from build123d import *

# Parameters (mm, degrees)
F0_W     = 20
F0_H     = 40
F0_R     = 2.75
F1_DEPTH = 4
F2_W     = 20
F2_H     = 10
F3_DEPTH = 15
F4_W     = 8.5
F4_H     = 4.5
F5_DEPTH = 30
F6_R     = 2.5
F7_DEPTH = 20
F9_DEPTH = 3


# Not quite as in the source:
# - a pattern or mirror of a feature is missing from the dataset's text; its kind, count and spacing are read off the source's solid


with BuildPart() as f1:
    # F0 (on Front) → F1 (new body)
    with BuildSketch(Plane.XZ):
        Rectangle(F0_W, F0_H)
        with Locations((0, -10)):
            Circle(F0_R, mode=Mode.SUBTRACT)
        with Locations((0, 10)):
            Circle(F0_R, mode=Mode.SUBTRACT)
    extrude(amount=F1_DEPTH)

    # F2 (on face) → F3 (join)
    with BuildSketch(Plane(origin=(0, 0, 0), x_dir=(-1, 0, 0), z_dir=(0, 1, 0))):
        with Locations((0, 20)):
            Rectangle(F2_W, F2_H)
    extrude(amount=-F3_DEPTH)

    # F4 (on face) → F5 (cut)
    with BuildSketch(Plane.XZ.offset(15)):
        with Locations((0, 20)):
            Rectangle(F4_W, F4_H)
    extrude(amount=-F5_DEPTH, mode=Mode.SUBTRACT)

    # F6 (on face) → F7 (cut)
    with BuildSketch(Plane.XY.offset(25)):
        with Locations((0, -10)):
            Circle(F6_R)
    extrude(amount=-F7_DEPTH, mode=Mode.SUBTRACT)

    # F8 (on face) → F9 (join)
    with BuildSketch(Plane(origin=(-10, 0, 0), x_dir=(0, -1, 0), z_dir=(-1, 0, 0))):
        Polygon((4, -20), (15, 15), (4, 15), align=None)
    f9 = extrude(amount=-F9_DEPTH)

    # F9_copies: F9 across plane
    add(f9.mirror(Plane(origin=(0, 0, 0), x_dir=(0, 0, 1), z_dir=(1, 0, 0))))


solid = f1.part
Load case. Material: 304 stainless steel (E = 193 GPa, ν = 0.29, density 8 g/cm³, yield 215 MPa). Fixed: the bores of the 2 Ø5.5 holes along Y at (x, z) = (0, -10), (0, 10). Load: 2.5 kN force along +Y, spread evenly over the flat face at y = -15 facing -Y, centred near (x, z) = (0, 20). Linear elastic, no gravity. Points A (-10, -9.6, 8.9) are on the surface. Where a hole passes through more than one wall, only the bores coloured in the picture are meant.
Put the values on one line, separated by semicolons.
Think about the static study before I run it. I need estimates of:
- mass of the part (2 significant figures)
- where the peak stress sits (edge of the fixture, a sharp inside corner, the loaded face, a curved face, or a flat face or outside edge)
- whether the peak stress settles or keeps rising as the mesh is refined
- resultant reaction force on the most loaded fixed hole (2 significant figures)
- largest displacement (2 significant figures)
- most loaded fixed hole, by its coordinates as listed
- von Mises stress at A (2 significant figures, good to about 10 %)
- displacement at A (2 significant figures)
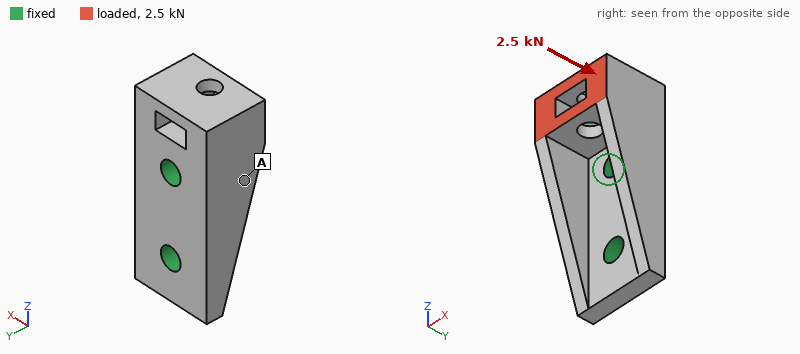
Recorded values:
49 g; edge of the fixture; keeps rising; 3.2 kN; 23 µm; (0, 10); 41 MPa; 6.1 µm
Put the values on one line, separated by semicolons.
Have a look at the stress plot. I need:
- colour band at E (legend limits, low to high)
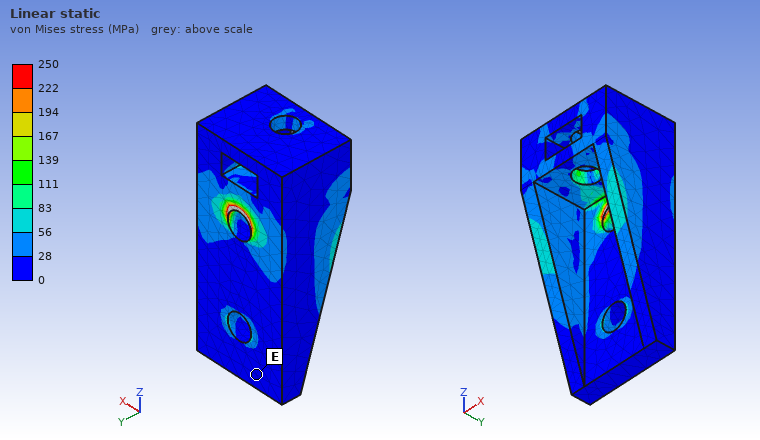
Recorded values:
0 to 28 MPa
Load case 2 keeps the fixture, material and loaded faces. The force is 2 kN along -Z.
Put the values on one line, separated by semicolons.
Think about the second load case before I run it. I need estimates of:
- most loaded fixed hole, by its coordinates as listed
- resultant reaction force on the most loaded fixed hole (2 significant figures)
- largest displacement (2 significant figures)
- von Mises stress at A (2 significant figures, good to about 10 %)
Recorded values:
(0, -10); 1.6 kN; 25 µm; 53 MPa
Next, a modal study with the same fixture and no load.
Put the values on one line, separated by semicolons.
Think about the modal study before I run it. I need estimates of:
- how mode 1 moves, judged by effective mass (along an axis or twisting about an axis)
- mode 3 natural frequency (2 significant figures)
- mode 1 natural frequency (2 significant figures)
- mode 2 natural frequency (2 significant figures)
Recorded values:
along X; 20 kHz; 10 kHz; 13 kHz
